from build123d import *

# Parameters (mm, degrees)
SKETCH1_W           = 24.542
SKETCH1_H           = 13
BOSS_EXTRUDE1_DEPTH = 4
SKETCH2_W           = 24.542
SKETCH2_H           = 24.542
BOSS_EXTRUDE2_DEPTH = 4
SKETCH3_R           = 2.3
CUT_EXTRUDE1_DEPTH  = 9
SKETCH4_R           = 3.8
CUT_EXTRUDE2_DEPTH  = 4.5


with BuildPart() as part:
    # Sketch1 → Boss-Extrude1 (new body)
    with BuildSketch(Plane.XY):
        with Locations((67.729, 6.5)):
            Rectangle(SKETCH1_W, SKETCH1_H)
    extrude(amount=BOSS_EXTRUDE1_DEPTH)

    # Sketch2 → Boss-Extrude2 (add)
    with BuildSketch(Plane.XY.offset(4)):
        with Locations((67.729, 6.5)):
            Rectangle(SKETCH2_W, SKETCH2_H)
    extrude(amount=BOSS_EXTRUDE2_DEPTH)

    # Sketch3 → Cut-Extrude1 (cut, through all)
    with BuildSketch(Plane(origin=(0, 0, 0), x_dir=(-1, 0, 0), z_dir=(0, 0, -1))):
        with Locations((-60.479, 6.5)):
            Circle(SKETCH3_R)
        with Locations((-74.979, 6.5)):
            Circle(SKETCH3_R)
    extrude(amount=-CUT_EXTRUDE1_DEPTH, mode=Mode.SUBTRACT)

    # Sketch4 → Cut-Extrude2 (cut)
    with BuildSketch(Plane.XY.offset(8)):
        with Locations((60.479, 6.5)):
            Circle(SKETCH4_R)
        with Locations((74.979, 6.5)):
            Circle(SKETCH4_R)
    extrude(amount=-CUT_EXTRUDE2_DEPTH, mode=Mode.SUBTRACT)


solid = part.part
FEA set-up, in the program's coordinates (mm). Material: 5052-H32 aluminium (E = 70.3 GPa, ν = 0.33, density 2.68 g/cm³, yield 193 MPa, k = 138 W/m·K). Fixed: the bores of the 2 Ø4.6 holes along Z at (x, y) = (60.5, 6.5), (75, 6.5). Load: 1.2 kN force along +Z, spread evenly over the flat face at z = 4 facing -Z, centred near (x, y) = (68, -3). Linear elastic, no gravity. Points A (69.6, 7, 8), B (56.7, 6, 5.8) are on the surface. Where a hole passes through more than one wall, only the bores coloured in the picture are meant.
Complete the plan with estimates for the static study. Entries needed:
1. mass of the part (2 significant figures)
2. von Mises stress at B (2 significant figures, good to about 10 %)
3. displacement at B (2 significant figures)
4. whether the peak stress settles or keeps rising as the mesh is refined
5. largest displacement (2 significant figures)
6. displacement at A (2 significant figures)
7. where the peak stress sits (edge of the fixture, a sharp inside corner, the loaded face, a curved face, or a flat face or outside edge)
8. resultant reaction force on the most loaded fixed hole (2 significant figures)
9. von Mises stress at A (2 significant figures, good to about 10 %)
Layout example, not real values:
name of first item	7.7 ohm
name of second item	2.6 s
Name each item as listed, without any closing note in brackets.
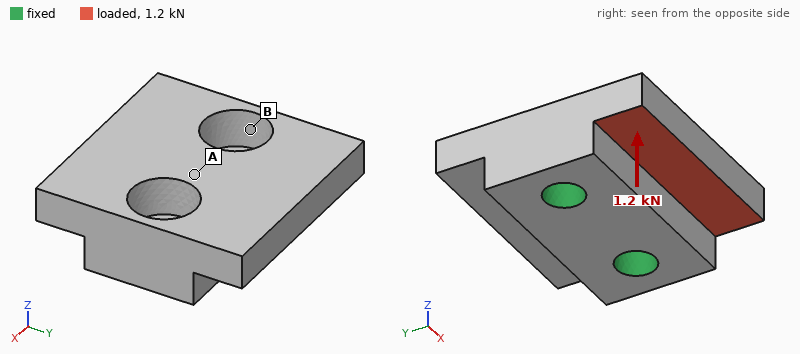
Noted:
mass of the part	8.5 g
von Mises stress at B	60 MPa
displacement at B	6.2 µm
whether the peak stress settles or keeps rising as the mesh is refined	keeps rising
largest displacement	37 µm
displacement at A	9.3 µm
where the peak stress sits	edge of the fixture
resultant reaction force on the most loaded fixed hole	610 N
von Mises stress at A	25 MPa
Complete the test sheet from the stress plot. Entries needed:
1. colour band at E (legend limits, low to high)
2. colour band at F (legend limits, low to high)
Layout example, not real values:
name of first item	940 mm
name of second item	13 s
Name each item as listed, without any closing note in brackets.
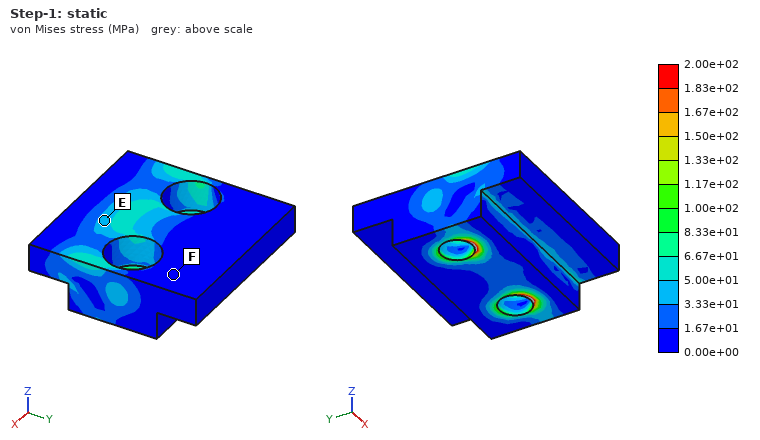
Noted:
colour band at E	3.33e+01 to 5.00e+01 MPa
colour band at F	0.00e+00 to 1.67e+01 MPa
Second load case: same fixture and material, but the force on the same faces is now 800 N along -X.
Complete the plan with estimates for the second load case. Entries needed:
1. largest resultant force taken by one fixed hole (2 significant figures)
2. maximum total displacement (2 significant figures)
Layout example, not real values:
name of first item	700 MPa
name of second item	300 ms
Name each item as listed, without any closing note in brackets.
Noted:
largest resultant force taken by one fixed hole	560 N
maximum total displacement	9.1 µm
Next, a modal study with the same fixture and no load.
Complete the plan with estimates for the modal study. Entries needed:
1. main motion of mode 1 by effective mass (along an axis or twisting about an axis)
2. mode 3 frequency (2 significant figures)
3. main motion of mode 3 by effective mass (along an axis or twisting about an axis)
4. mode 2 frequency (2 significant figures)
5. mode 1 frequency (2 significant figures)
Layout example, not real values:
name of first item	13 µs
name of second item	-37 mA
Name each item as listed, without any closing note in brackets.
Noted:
main motion of mode 1 by effective mass	along Y
mode 3 frequency	34 kHz
main motion of mode 3 by effective mass	along Z
mode 2 frequency	32 kHz
mode 1 frequency	19 kHz
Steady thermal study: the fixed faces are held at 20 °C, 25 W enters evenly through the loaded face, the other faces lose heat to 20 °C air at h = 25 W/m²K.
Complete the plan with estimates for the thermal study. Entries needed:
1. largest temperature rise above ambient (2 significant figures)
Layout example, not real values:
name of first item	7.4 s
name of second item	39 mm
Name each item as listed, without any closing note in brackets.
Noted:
largest temperature rise above ambient	18 K
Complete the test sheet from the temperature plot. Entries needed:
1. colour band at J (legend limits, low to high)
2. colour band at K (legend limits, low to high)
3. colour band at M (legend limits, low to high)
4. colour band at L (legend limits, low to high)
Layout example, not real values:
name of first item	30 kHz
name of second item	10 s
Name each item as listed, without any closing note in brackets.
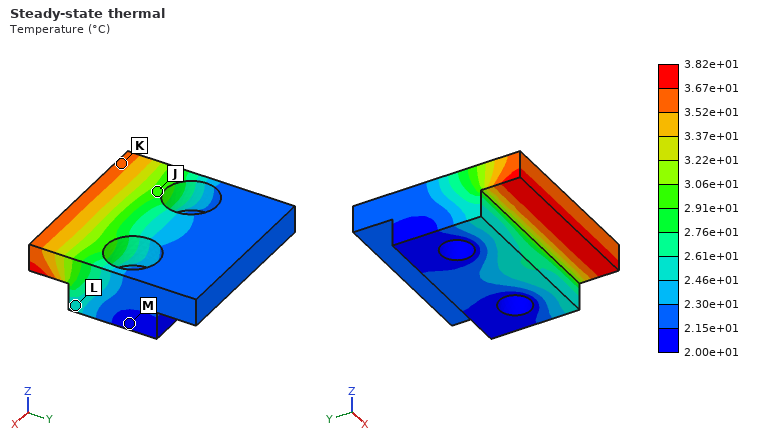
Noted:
colour band at J	2.91e+01 to 3.06e+01 °C
colour band at K	3.52e+01 to 3.67e+01 °C
colour band at M	2.00e+01 to 2.15e+01 °C
colour band at L	2.46e+01 to 2.61e+01 °C
